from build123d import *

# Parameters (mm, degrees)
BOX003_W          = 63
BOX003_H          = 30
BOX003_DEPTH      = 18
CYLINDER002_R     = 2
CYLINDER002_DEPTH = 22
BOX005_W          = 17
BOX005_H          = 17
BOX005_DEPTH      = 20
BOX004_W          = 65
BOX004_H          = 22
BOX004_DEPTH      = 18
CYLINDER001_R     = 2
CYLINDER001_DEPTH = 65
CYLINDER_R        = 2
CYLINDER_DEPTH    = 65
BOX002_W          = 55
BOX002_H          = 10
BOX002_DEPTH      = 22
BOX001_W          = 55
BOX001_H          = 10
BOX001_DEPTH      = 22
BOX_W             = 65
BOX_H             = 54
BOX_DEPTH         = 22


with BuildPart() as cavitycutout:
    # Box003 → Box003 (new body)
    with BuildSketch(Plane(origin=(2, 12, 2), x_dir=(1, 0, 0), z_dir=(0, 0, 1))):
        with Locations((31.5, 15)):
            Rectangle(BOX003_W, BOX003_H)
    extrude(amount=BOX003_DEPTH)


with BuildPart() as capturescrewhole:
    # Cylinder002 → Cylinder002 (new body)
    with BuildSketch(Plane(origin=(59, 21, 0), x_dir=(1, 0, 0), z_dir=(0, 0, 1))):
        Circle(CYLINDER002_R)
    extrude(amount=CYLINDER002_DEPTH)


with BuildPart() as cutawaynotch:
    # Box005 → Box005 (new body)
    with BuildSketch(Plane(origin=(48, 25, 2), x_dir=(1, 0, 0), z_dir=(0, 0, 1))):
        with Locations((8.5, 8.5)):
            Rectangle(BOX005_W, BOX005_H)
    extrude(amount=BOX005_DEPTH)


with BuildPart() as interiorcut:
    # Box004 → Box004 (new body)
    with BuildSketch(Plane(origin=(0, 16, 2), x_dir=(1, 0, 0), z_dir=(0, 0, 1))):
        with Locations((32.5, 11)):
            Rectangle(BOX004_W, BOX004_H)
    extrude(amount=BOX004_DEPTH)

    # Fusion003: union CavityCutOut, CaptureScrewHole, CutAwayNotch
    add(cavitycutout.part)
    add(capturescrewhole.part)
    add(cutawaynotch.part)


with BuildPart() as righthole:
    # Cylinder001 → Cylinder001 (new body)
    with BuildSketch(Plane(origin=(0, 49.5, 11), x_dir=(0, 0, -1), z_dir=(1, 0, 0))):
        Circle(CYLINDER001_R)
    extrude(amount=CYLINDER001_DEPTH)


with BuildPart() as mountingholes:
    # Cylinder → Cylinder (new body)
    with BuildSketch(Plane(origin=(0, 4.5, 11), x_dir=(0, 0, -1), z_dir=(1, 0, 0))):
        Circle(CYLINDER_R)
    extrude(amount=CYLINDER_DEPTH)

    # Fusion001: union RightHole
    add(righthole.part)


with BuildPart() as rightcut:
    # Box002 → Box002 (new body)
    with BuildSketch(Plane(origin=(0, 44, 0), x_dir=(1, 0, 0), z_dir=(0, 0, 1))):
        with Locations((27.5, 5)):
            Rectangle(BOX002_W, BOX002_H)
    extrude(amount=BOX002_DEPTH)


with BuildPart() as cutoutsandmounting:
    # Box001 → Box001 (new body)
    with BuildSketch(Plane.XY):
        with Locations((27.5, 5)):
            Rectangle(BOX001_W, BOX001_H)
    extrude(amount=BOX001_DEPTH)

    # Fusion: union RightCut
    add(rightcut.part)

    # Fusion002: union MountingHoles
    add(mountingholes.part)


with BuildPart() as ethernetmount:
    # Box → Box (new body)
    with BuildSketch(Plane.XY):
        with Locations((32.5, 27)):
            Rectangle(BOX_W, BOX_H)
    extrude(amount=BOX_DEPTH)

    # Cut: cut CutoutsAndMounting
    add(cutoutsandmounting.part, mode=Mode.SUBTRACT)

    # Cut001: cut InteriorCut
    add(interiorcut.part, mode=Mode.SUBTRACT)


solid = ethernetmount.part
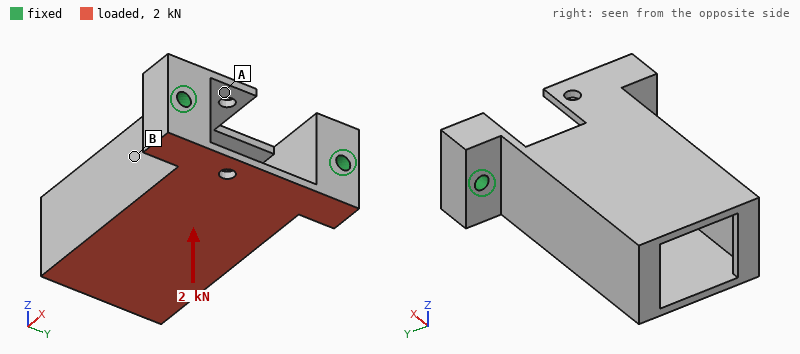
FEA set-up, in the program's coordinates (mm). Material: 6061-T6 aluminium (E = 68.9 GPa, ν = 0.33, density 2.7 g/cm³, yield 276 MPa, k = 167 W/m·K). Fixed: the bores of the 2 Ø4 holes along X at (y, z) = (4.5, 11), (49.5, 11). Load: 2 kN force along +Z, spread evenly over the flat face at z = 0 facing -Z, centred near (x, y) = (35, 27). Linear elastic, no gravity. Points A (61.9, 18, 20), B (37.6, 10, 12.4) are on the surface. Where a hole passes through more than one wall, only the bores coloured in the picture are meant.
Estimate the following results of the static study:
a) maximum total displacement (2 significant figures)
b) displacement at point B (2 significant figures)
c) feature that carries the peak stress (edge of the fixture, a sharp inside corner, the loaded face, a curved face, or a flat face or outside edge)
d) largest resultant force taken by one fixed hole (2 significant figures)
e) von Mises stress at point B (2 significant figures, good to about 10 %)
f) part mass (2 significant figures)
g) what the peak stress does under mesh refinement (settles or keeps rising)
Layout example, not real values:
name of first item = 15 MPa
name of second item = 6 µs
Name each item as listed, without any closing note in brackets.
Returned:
maximum total displacement = 0.26 mm
displacement at point B = 0.076 mm
feature that carries the peak stress = edge of the fixture
largest resultant force taken by one fixed hole = 1.1 kN
von Mises stress at point B = 32 MPa
part mass = 47 g
what the peak stress does under mesh refinement = keeps rising
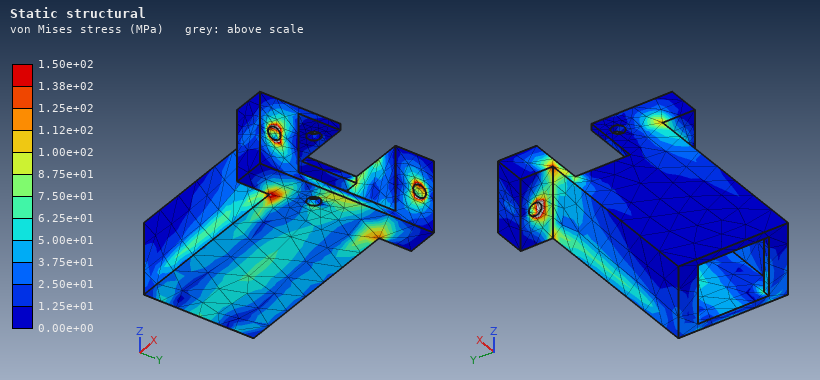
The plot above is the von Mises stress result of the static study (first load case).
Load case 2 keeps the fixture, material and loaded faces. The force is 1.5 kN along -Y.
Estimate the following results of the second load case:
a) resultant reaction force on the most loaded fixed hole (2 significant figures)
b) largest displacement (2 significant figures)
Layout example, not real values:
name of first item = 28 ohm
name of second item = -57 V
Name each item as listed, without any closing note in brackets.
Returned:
resultant reaction force on the most loaded fixed hole = 1.3 kN
largest displacement = 59 µm
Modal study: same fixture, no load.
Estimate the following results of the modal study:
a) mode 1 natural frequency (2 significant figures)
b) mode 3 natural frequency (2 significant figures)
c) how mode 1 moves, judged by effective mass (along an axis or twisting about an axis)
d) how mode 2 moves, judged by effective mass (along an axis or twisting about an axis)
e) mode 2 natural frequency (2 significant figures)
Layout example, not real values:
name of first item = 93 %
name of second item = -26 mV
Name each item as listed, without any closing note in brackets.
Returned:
mode 1 natural frequency = 2700 Hz
mode 3 natural frequency = 5600 Hz
how mode 1 moves, judged by effective mass = along Z
how mode 2 moves, judged by effective mass = along Y
mode 2 natural frequency = 5300 Hz
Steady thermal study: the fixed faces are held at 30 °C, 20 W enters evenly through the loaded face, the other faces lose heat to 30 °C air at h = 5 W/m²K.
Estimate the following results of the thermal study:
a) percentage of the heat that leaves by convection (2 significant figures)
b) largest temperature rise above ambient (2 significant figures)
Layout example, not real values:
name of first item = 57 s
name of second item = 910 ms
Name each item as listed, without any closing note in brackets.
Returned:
percentage of the heat that leaves by convection = 3.6 %
largest temperature rise above ambient = 21 K
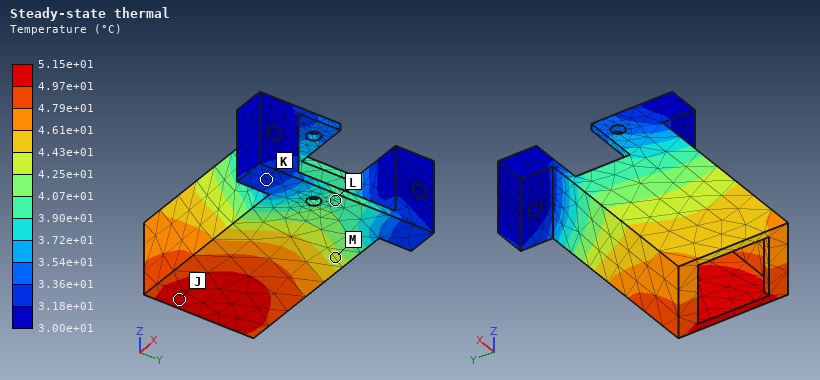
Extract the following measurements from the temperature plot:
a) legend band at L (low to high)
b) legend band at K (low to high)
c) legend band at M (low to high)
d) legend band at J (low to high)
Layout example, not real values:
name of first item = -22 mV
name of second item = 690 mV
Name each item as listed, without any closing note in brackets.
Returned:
legend band at L = 3.90e+01 to 4.07e+01 °C
legend band at K = 3.18e+01 to 3.36e+01 °C
legend band at M = 4.25e+01 to 4.43e+01 °C
legend band at J = 4.97e+01 to 5.15e+01 °C
